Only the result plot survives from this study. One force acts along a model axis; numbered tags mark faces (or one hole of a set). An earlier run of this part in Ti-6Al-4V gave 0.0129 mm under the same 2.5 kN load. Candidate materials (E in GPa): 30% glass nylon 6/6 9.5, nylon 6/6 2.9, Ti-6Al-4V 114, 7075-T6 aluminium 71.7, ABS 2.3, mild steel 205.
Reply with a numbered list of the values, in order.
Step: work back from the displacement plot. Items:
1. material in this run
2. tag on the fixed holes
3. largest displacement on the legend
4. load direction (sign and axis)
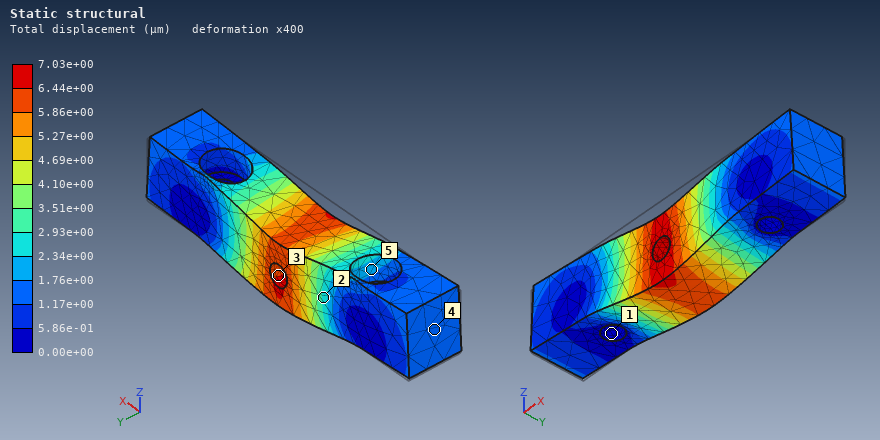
1. mild steel
2. 1
3. 7.03e+00 µm
4. -Z
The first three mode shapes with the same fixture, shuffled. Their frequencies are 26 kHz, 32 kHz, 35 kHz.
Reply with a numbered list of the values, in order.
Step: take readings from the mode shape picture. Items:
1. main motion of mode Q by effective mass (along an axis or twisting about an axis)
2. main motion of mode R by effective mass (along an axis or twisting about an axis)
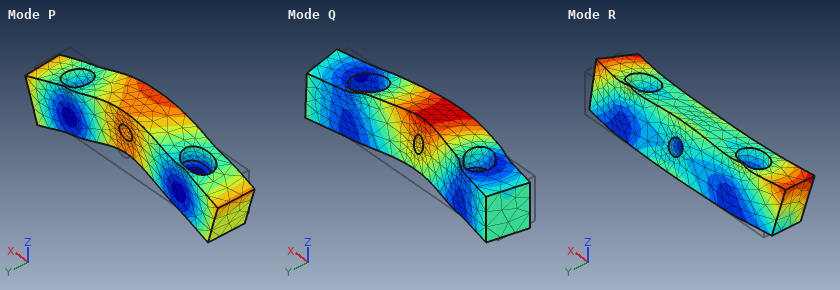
1. along Y
2. along Y
